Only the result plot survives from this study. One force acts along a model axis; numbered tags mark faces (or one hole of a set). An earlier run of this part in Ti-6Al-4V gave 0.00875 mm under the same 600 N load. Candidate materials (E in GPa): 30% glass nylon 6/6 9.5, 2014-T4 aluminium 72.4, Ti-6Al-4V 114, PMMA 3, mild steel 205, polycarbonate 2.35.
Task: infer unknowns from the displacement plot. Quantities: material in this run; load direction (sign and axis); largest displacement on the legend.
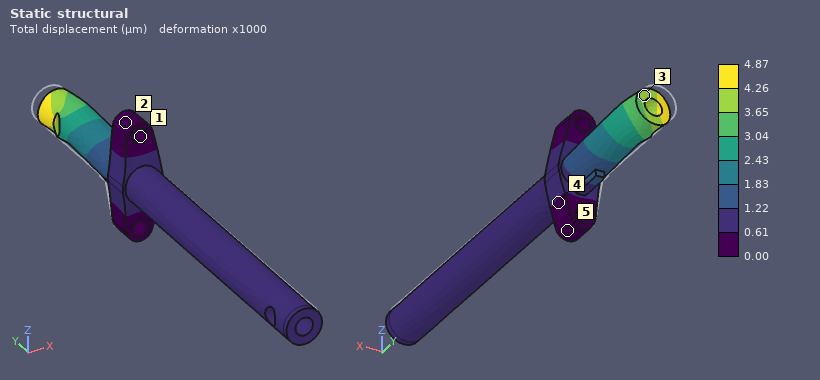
mild steel
-Y
4.87 µm
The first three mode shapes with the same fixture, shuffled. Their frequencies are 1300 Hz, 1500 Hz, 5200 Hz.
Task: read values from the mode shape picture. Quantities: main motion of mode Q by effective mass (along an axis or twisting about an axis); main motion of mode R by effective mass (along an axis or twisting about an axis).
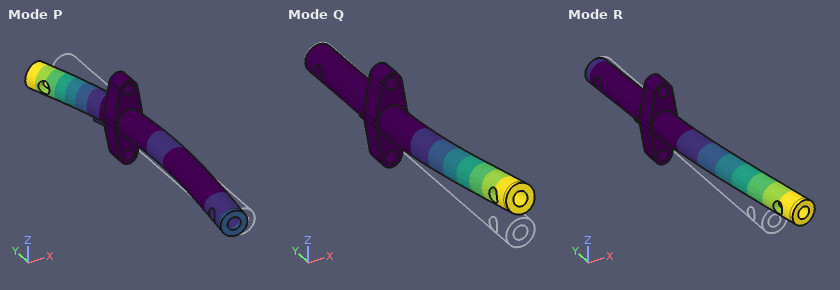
along Z
along X
